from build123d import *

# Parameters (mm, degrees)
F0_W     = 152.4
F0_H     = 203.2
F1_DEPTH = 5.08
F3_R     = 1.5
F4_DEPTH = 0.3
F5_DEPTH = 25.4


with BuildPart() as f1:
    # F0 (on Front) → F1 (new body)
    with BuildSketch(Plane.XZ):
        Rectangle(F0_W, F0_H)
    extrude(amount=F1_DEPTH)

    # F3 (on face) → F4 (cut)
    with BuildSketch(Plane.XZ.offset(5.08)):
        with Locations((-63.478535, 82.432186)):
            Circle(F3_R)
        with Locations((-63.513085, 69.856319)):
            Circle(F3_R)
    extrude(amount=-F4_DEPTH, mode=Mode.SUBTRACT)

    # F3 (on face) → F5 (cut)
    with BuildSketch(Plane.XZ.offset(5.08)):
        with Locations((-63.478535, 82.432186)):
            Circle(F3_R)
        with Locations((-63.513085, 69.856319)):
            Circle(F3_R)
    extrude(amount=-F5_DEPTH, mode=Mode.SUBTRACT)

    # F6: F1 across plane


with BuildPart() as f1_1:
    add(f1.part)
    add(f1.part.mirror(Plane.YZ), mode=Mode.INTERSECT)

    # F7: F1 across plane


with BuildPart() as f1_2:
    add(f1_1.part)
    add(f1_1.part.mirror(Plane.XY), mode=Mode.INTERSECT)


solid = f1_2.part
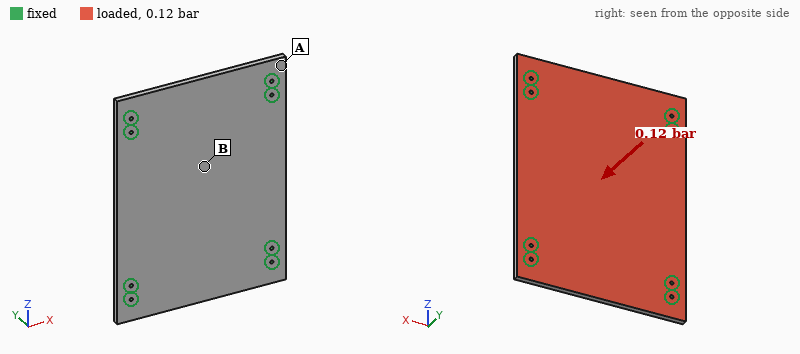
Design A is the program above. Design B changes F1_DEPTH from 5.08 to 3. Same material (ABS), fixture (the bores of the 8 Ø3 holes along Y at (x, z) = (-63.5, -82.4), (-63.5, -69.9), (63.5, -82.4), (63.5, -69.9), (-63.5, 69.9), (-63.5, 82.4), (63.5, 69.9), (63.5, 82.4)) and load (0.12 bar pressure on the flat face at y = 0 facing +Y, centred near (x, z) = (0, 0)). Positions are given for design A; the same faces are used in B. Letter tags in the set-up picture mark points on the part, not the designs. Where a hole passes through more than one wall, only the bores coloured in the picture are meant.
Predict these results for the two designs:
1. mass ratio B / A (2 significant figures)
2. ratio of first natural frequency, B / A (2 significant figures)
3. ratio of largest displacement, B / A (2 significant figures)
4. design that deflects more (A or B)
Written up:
0.59
0.61
4.6
B
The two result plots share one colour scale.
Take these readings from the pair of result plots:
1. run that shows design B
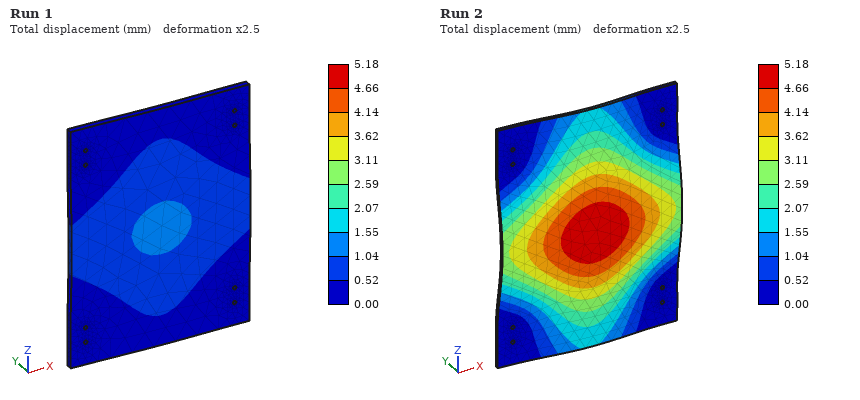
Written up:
Run 2
